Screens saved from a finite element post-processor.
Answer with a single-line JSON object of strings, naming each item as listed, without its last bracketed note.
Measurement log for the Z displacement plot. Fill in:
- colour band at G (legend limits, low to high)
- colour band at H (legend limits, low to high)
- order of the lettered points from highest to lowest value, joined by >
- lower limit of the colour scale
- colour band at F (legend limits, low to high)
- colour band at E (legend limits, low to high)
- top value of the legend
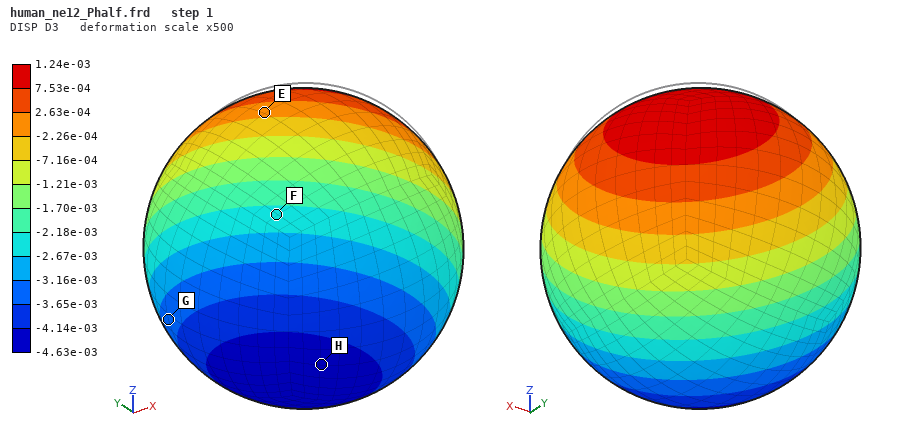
{"colour band at G": "-3.65e-03 to -3.16e-03", "colour band at H": "-4.63e-03 to -4.14e-03", "order of the lettered points from highest to lowest value, joined by >": "E > F > G > H", "lower limit of the colour scale": "-4.63e-03", "colour band at F": "-2.67e-03 to -2.18e-03", "colour band at E": "-2.26e-04 to 2.63e-04", "top value of the legend": "1.24e-03"}
